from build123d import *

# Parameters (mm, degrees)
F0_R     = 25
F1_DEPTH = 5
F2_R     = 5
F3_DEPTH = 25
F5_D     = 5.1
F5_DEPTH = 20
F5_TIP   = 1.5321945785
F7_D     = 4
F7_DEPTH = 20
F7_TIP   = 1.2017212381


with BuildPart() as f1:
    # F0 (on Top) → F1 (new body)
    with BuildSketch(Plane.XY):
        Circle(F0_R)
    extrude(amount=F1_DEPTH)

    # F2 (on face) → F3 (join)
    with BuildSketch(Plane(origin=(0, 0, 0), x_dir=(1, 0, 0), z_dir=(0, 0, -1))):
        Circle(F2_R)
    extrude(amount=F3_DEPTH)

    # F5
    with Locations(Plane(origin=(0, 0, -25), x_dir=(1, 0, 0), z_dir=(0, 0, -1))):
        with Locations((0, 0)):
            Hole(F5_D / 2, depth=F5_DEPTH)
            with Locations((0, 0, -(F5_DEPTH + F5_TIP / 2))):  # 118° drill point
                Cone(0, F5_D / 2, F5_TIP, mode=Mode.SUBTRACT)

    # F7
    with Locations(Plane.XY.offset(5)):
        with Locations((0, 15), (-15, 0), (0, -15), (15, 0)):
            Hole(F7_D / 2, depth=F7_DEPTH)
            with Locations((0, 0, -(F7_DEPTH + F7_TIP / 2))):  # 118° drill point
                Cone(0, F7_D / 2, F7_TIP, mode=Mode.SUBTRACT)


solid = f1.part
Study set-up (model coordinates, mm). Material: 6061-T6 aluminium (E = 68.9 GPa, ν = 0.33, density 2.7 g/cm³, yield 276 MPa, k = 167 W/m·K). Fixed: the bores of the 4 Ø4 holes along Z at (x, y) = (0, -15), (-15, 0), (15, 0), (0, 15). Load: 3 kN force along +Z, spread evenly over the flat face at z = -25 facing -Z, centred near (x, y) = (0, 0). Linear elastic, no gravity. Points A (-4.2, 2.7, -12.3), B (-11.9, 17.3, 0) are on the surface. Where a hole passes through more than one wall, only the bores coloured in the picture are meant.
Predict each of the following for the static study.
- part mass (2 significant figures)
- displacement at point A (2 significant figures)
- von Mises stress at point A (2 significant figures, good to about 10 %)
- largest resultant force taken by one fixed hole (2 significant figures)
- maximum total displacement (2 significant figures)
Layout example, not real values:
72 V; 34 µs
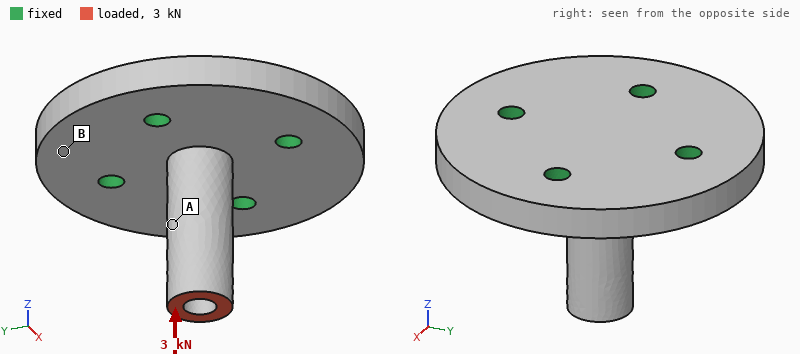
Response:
30 g; 24 µm; 52 MPa; 760 N; 33 µm
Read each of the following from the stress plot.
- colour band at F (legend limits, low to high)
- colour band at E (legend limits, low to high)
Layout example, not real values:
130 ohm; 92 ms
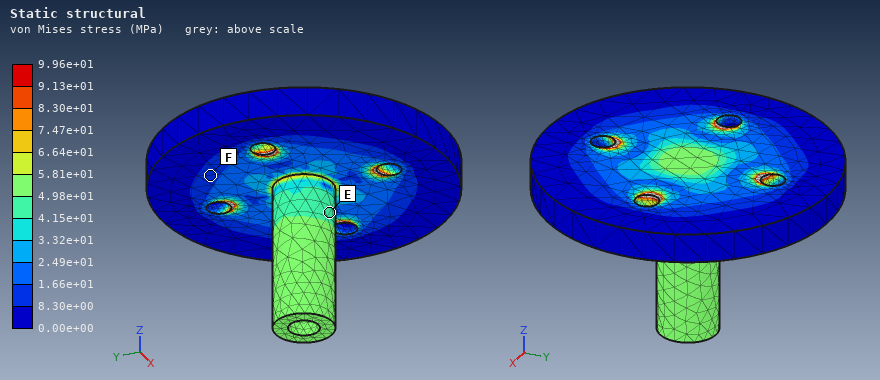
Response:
8.30e+00 to 1.66e+01 MPa; 4.15e+01 to 4.98e+01 MPa
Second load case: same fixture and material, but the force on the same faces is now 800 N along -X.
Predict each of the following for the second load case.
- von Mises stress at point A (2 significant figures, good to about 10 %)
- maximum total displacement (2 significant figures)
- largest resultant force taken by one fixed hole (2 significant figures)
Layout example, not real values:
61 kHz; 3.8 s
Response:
96 MPa; 0.23 mm; 910 N
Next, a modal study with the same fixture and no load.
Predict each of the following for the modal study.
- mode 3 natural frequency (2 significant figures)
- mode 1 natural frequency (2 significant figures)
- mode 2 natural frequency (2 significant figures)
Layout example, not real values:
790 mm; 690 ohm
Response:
20 kHz; 8900 Hz; 8900 Hz
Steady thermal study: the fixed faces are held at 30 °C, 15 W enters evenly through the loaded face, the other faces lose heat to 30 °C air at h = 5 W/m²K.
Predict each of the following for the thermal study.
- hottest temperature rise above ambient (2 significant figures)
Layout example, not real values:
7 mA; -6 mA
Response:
42 K
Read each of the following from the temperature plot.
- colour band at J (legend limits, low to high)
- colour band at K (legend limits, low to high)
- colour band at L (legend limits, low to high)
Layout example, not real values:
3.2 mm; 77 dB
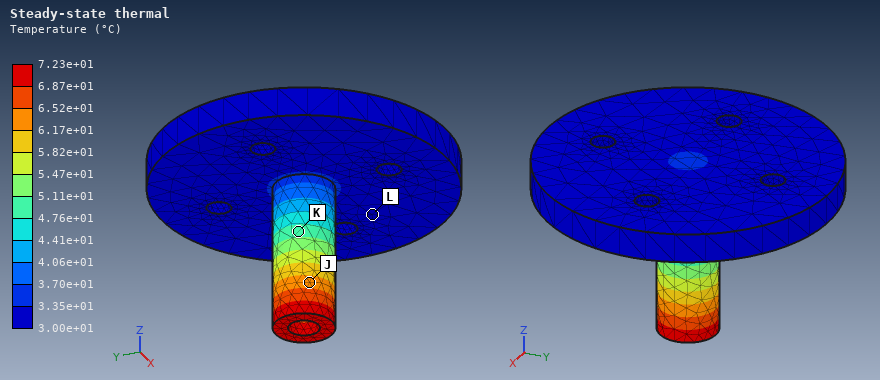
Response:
6.17e+01 to 6.52e+01 °C; 4.76e+01 to 5.11e+01 °C; 3.00e+01 to 3.35e+01 °C
